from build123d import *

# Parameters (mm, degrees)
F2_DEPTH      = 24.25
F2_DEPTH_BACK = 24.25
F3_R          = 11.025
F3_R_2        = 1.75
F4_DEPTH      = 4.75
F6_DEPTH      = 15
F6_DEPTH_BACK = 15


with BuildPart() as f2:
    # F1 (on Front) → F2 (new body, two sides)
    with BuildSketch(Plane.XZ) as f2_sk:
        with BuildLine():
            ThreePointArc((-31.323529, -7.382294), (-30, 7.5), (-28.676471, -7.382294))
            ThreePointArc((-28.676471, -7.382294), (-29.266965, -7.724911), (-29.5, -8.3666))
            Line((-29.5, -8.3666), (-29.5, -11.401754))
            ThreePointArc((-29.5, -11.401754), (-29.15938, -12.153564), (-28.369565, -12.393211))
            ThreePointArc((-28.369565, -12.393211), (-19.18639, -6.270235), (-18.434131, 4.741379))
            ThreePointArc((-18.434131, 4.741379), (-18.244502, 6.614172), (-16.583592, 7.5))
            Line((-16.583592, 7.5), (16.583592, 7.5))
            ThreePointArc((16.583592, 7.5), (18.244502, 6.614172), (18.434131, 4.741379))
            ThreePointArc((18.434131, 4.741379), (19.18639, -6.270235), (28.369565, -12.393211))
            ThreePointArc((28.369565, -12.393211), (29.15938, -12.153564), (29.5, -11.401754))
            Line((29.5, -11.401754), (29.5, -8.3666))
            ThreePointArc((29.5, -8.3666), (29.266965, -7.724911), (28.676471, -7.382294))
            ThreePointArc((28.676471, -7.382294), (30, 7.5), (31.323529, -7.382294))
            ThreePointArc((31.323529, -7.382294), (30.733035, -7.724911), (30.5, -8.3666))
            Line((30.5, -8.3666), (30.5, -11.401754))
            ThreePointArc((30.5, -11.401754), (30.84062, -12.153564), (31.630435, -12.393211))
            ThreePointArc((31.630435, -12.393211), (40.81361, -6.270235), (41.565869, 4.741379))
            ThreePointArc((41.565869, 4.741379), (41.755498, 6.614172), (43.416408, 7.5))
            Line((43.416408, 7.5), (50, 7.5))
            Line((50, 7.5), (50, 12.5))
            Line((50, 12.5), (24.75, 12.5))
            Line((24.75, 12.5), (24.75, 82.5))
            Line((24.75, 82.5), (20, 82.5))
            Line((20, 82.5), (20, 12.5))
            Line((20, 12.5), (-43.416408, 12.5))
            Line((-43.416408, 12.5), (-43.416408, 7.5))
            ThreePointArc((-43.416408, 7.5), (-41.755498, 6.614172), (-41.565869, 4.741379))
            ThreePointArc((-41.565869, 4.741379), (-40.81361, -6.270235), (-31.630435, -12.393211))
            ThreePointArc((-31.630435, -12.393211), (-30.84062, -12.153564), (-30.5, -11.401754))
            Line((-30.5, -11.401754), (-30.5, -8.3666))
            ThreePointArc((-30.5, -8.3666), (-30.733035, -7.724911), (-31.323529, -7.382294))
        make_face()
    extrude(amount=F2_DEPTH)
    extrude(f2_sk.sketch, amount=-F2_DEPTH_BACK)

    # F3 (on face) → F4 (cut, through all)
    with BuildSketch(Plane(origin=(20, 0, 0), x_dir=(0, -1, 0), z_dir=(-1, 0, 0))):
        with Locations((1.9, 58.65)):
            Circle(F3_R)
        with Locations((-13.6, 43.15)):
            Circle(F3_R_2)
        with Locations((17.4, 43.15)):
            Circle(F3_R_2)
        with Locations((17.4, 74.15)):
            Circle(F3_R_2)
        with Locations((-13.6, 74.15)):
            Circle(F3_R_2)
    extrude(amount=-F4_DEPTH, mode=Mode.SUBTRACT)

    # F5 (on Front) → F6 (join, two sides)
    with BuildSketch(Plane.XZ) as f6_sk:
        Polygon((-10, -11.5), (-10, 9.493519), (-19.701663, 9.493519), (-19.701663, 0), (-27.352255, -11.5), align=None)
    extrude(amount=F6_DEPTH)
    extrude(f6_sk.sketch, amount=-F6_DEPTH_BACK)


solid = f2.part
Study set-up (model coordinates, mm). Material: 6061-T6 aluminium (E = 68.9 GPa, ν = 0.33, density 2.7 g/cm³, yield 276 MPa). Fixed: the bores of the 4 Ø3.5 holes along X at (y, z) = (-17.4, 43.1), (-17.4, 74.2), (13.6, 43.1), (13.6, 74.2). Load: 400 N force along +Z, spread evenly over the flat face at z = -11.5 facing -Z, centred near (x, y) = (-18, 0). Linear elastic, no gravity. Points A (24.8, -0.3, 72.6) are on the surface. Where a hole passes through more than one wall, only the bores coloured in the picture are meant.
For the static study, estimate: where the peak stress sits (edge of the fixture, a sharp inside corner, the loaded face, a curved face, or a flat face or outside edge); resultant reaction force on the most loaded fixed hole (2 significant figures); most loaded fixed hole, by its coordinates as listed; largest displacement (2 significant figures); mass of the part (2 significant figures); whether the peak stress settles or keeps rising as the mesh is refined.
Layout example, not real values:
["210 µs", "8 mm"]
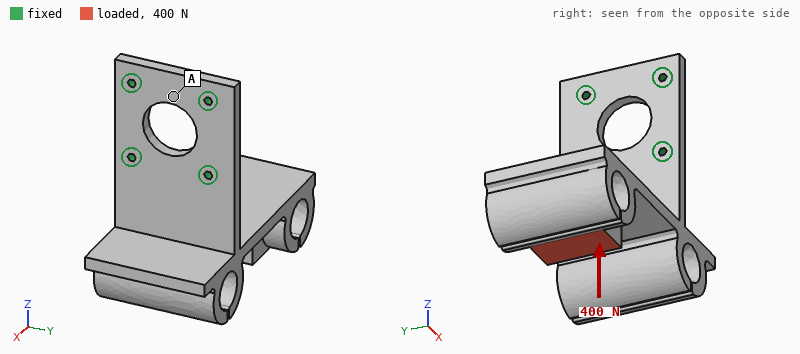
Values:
["edge of the fixture", "210 N", "(13.6, 43.1)", "1.6 mm", "180 g", "keeps rising"]
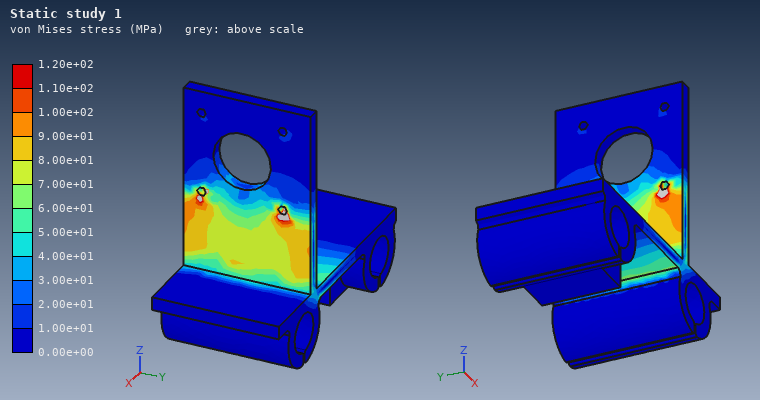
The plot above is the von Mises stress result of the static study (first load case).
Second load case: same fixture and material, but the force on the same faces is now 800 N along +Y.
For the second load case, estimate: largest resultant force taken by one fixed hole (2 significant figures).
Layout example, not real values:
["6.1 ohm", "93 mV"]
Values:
["1.6 kN"]
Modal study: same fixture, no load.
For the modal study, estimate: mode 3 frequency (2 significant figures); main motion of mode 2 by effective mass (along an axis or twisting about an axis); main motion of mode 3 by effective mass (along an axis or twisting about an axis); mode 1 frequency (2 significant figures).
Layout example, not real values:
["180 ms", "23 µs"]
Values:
["1000 Hz", "along Y", "along X", "270 Hz"]
